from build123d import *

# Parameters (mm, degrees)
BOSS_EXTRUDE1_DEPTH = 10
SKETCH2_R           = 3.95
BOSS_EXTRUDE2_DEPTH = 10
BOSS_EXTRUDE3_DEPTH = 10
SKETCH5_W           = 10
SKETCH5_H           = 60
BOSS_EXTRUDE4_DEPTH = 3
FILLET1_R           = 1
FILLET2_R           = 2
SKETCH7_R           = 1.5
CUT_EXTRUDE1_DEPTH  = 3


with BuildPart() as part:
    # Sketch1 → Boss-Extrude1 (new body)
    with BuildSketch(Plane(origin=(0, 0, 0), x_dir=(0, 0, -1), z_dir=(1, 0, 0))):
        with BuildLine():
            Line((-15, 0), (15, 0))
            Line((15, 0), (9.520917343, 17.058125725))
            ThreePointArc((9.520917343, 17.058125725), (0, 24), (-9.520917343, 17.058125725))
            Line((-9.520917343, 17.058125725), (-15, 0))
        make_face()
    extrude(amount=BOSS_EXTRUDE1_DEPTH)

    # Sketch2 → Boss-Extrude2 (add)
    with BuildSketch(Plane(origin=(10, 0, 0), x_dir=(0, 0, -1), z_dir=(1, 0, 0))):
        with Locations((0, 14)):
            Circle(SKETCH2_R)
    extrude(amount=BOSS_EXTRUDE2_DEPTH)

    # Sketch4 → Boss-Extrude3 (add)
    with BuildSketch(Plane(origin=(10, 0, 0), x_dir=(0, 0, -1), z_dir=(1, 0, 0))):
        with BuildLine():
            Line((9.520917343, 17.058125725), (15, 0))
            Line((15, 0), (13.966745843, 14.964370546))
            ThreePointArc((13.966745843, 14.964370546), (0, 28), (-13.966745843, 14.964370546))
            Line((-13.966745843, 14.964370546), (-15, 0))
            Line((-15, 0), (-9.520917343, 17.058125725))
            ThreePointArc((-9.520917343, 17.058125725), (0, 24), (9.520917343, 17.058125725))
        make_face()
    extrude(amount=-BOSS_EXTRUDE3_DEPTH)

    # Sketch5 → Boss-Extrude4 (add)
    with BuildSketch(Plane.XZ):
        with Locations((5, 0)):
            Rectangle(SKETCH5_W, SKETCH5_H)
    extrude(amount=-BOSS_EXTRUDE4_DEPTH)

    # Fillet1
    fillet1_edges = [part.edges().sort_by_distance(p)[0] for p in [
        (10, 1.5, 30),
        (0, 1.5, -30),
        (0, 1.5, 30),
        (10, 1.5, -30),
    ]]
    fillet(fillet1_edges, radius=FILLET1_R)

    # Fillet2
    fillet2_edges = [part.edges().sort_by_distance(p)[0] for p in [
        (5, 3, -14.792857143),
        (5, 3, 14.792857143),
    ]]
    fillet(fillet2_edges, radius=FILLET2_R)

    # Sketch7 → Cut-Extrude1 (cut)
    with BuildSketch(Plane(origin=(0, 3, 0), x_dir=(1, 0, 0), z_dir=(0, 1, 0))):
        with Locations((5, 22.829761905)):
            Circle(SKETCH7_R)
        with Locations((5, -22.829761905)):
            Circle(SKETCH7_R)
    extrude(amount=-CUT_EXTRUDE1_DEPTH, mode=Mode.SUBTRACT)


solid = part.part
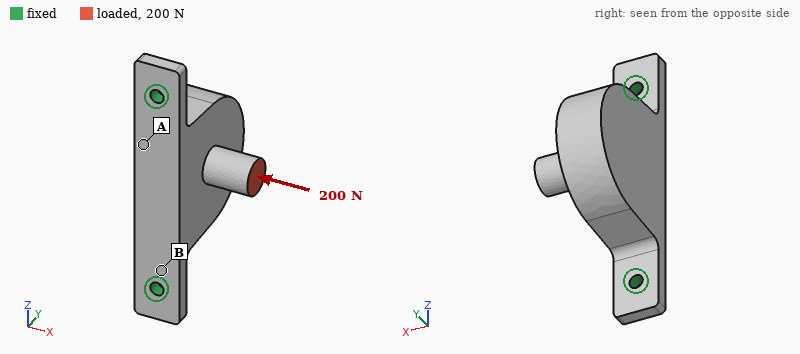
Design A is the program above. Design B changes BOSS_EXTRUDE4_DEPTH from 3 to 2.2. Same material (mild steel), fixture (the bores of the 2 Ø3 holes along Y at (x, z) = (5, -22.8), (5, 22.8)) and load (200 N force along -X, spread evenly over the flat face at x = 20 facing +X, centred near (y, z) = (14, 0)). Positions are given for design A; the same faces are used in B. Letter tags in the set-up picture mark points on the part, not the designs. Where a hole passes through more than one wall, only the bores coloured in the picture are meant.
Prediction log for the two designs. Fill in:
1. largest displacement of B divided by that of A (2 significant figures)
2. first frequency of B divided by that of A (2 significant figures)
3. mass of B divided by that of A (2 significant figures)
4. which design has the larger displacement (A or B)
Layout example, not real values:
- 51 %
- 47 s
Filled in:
- 2.1
- 0.69
- 0.97
- B
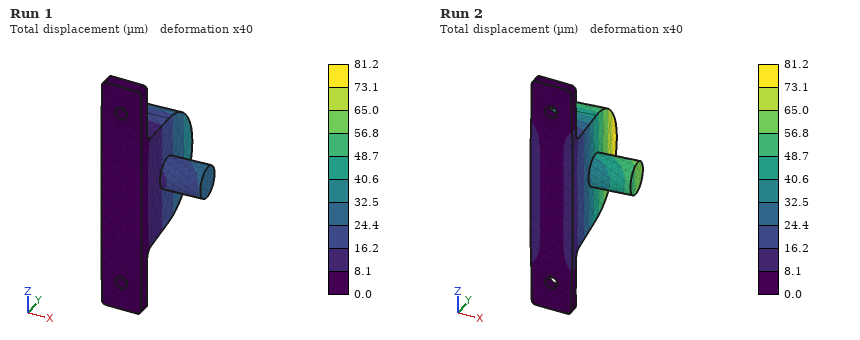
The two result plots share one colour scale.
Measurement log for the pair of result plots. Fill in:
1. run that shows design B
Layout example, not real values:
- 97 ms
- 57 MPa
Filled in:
- Run 2
